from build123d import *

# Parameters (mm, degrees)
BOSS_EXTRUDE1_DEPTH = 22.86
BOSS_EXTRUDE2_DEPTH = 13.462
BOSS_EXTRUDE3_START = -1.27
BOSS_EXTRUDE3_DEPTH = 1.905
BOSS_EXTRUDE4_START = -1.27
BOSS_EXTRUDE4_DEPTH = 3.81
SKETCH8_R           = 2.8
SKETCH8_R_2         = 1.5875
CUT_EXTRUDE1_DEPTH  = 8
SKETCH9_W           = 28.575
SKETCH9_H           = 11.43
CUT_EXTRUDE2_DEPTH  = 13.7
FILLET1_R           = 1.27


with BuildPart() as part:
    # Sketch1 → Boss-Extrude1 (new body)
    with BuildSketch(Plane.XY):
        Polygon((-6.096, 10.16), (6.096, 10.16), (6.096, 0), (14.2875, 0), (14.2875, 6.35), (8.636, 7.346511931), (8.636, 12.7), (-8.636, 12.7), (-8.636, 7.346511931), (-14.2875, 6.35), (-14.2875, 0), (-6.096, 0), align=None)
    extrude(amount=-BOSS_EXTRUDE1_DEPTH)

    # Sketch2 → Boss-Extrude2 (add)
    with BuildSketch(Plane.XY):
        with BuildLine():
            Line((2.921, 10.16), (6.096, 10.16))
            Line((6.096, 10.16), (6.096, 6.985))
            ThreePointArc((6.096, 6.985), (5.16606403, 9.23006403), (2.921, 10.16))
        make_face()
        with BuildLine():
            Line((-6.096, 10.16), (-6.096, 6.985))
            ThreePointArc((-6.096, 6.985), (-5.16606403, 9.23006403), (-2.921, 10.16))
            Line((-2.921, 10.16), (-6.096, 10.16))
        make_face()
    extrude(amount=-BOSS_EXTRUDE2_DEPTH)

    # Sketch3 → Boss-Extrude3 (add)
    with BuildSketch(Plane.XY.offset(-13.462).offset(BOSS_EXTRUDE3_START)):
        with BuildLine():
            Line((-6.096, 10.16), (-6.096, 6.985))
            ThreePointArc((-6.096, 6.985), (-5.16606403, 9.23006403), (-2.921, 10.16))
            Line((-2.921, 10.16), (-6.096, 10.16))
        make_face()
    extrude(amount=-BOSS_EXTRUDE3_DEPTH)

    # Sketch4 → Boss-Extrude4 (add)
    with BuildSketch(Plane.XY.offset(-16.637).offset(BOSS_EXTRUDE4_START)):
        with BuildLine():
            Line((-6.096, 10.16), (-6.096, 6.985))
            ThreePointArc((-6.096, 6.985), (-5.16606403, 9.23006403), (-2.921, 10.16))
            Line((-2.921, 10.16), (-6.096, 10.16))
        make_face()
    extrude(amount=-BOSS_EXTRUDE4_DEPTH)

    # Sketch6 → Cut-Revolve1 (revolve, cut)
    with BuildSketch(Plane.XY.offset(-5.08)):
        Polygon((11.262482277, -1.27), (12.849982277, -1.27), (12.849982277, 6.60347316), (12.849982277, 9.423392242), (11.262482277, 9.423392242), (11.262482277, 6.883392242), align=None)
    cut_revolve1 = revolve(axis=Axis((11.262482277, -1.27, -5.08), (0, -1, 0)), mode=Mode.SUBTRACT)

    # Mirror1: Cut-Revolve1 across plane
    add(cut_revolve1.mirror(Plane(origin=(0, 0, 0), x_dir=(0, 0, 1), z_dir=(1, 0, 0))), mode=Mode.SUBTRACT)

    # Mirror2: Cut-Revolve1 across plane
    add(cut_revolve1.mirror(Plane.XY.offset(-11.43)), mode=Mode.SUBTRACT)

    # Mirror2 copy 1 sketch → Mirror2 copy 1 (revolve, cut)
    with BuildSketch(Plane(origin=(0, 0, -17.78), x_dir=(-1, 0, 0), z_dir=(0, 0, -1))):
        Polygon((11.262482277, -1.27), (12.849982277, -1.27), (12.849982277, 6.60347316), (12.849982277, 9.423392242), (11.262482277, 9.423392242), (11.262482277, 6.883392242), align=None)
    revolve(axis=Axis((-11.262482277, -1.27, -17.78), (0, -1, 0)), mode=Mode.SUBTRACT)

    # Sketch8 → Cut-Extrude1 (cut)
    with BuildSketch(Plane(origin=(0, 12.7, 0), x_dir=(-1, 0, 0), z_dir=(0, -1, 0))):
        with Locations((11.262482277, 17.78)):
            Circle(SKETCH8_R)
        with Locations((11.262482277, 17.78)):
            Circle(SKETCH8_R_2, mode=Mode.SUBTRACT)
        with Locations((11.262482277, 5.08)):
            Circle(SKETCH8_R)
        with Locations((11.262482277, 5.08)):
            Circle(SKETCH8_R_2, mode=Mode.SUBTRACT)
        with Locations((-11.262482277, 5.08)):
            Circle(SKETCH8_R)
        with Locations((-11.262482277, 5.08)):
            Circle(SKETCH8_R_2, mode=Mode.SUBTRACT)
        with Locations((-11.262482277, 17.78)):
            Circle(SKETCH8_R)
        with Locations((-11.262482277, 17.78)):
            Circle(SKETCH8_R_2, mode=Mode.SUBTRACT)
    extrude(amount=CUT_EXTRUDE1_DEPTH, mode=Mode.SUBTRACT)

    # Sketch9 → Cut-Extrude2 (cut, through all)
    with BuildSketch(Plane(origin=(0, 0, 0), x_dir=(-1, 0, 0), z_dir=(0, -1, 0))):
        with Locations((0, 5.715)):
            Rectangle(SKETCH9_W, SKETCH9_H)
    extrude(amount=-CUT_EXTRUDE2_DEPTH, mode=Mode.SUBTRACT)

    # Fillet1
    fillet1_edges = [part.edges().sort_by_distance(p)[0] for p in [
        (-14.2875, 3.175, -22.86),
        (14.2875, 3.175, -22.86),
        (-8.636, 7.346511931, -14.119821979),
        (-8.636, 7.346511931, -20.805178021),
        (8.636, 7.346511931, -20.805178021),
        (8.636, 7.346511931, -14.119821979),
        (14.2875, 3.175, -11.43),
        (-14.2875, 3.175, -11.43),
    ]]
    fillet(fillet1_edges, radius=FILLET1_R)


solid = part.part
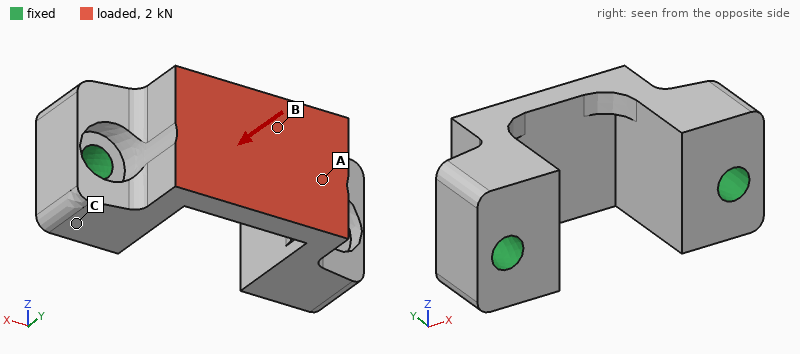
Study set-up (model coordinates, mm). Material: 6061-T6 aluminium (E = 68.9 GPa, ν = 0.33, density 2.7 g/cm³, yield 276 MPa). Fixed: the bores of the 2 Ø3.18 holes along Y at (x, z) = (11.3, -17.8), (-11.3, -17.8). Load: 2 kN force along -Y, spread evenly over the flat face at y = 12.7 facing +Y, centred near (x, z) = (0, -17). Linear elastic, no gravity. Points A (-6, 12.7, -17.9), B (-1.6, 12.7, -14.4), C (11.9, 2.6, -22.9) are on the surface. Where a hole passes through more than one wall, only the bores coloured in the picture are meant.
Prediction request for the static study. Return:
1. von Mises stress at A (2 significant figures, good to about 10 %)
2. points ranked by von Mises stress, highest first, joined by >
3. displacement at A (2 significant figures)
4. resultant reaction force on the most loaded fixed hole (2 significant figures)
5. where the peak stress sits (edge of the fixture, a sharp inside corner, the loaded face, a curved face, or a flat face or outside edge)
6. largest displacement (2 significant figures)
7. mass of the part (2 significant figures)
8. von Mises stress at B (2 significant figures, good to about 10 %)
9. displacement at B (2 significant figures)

24 MPa
B > A > C
10 µm
1.1 kN
a curved face
22 µm
4.9 g
68 MPa
19 µm
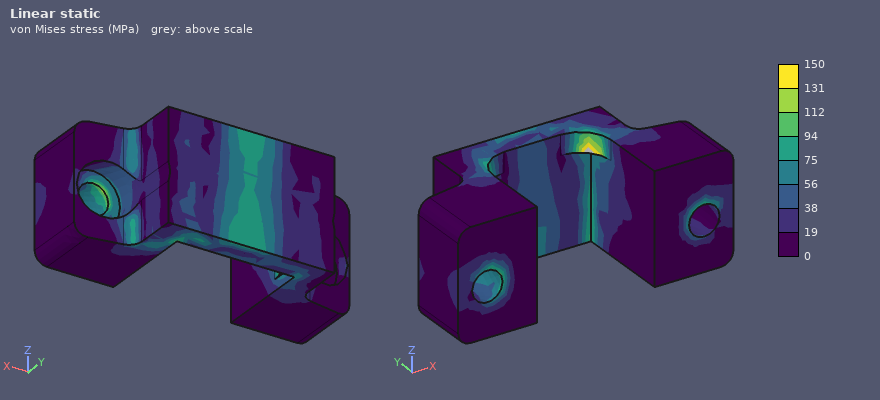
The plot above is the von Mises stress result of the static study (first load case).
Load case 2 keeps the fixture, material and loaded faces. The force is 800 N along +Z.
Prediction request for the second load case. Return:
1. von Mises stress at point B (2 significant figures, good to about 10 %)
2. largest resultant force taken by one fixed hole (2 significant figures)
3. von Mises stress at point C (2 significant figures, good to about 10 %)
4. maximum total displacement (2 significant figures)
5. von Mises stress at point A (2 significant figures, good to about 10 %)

13 MPa
410 N
26 MPa
28 µm
25 MPa
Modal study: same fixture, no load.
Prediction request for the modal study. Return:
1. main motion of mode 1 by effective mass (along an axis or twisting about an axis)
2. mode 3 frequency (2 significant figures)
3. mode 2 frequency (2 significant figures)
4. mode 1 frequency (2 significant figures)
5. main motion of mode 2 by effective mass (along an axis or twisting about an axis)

along Z
35 kHz
29 kHz
24 kHz
along X
